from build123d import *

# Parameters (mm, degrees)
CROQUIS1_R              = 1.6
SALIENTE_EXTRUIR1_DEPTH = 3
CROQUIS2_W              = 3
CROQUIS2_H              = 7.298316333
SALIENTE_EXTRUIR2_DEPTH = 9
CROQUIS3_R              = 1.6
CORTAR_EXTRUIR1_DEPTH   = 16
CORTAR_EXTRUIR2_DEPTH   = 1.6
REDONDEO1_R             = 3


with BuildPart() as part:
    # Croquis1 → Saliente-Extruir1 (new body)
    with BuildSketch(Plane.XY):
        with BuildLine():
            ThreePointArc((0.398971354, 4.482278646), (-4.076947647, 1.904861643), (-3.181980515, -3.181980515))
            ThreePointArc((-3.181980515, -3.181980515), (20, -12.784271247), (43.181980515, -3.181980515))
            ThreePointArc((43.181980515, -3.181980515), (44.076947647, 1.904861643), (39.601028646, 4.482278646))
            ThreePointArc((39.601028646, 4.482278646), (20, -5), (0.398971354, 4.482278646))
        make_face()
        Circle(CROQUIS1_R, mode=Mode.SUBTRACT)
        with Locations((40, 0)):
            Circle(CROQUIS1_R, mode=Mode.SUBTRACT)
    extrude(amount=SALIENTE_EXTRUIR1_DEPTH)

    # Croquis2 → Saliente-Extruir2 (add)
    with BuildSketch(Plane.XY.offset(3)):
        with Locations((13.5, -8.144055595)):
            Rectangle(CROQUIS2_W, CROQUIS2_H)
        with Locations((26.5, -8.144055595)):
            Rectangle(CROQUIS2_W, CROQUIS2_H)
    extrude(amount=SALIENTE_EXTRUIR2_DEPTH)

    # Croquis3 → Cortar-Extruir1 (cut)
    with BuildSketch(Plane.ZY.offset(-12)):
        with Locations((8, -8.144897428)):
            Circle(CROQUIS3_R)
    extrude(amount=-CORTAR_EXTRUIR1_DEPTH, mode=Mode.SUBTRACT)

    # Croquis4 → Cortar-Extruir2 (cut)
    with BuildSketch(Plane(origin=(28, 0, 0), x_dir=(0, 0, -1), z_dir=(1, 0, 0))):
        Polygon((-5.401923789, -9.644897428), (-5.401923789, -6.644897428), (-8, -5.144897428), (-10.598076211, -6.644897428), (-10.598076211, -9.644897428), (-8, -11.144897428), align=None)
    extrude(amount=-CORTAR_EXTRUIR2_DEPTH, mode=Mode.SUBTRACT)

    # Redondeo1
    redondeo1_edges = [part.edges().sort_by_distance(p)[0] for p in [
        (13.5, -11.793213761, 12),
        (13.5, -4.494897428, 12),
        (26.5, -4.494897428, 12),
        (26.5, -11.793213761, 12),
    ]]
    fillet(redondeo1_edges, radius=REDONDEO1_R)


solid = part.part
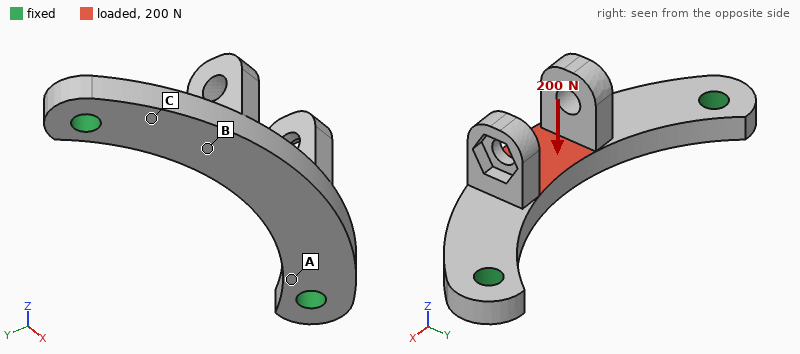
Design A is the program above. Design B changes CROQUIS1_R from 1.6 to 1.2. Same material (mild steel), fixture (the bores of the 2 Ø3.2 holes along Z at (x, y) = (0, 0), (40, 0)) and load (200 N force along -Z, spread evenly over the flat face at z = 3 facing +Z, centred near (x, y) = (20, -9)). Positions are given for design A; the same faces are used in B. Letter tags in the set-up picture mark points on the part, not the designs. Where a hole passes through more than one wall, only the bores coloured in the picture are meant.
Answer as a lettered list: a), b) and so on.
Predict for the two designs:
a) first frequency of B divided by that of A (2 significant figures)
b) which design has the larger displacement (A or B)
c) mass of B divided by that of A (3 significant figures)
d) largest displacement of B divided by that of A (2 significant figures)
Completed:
a) 0.95
b) B
c) 1.01
d) 1.1
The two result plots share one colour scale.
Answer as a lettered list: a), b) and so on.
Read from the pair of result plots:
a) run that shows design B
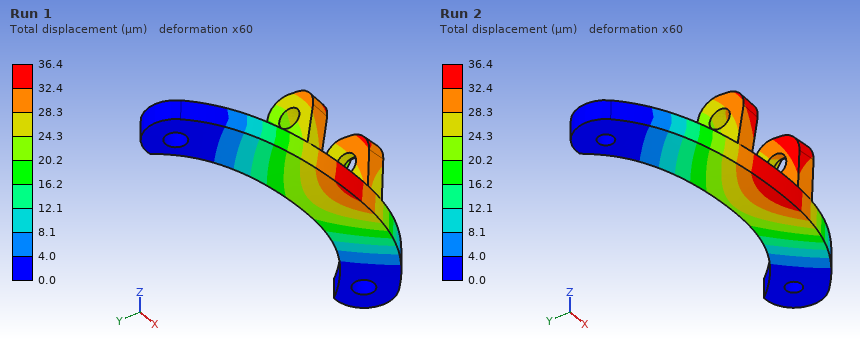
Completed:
a) Run 2
